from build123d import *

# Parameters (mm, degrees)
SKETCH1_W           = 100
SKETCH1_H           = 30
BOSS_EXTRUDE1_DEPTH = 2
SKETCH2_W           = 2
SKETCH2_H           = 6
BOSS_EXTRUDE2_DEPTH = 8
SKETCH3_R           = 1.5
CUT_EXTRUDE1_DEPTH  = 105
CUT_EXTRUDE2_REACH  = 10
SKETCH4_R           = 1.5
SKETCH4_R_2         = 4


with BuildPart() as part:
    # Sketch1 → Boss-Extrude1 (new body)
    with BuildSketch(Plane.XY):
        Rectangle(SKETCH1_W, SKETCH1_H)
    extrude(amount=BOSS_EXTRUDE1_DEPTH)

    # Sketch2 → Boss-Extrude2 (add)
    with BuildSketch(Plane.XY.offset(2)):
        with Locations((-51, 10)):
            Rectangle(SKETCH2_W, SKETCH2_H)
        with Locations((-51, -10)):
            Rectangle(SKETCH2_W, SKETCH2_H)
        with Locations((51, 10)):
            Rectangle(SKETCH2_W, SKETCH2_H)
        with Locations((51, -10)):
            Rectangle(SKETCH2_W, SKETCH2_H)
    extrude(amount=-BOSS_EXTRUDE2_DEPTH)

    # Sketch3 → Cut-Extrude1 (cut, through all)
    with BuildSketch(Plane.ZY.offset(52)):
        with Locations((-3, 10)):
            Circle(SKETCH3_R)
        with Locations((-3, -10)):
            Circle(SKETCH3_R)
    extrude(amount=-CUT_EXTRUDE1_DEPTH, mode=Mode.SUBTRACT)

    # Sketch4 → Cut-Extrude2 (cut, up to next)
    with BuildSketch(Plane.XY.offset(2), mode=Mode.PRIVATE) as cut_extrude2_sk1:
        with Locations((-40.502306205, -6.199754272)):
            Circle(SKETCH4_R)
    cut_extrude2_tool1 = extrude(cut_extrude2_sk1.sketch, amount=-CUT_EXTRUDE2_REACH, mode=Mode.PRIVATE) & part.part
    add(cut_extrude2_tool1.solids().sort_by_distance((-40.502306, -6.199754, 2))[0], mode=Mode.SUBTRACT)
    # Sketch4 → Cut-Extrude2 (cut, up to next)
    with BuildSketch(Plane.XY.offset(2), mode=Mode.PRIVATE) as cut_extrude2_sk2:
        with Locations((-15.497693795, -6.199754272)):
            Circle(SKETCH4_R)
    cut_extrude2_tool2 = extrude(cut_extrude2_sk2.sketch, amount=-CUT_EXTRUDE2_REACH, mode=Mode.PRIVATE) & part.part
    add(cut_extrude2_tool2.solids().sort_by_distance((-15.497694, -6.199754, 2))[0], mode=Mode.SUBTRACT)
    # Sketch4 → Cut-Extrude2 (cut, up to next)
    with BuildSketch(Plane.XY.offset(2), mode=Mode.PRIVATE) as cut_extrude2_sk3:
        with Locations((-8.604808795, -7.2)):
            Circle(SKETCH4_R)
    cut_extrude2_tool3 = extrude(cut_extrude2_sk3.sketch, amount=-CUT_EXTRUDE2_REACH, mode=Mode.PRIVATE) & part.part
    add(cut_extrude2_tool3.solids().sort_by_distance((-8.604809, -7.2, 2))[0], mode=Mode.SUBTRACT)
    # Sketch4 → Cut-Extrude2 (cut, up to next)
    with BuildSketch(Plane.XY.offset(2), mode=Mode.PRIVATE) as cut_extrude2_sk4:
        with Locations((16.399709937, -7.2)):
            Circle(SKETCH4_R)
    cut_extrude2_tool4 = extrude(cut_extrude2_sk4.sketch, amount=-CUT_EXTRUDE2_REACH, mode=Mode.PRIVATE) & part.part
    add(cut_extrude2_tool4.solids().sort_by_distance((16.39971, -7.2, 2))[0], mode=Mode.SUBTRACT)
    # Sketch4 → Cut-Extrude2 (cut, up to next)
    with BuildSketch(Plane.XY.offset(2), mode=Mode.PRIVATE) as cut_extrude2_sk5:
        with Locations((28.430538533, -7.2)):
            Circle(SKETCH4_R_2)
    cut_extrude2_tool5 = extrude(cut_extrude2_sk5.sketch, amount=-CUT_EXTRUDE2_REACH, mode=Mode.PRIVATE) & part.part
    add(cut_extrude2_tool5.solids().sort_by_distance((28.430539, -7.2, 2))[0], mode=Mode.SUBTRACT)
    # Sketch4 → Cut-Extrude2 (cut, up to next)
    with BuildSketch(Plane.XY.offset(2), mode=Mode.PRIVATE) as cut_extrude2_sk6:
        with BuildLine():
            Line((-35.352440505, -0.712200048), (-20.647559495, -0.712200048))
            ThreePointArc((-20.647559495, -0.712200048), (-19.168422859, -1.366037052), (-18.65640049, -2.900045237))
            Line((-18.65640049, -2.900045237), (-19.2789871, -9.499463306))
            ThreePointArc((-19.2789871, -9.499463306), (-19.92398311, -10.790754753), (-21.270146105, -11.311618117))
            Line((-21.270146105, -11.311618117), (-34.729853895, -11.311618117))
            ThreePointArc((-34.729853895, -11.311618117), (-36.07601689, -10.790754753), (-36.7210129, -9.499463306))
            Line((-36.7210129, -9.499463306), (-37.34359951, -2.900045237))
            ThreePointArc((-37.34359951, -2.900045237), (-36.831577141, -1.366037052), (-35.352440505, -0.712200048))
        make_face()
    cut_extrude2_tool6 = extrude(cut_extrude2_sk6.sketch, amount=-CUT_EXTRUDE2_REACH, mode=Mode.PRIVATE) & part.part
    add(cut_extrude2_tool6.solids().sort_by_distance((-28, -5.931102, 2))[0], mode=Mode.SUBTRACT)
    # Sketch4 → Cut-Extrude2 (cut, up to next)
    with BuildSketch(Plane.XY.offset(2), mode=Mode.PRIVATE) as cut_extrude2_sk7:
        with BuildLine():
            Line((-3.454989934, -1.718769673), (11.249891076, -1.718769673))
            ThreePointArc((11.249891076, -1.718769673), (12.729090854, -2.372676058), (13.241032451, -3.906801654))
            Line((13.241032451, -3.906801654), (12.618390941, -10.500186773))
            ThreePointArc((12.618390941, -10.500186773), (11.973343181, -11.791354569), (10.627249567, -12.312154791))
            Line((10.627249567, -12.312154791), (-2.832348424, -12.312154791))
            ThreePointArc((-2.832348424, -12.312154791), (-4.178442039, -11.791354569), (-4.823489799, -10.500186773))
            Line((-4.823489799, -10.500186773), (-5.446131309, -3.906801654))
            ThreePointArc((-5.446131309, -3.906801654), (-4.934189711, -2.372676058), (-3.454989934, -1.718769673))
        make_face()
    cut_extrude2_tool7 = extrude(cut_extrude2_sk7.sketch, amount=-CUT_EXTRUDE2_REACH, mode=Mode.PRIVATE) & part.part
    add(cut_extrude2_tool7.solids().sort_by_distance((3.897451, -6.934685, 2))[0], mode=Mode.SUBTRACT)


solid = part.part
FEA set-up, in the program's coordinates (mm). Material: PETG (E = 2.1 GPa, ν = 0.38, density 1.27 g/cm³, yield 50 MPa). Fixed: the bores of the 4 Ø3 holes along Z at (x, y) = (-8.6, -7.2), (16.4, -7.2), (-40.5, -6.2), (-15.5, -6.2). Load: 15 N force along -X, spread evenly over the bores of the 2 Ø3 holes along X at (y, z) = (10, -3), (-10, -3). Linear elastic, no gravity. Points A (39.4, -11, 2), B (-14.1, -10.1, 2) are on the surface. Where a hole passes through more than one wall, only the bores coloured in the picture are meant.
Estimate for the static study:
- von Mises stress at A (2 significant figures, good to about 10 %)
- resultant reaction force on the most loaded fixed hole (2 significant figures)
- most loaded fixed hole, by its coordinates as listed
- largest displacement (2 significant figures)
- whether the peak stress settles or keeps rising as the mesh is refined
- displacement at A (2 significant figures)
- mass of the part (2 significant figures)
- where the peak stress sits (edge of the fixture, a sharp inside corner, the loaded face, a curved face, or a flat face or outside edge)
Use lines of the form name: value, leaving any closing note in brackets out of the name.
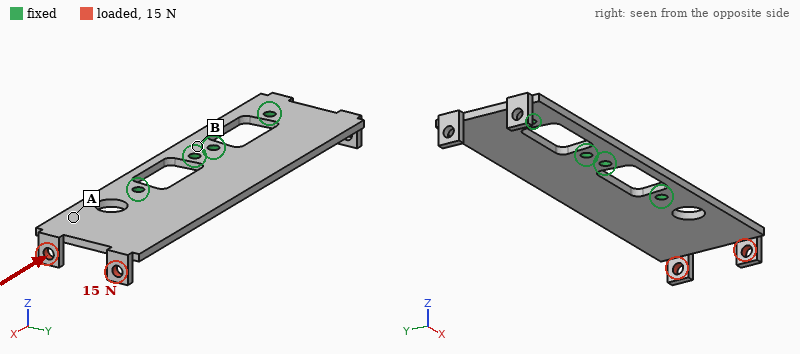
von Mises stress at A: 2.6 MPa
resultant reaction force on the most loaded fixed hole: 9.5 N
most loaded fixed hole, by its coordinates as listed: (16.4, -7.2)
largest displacement: 1.3 mm
whether the peak stress settles or keeps rising as the mesh is refined: keeps rising
displacement at A: 0.47 mm
mass of the part: 6.9 g
where the peak stress sits: edge of the fixture
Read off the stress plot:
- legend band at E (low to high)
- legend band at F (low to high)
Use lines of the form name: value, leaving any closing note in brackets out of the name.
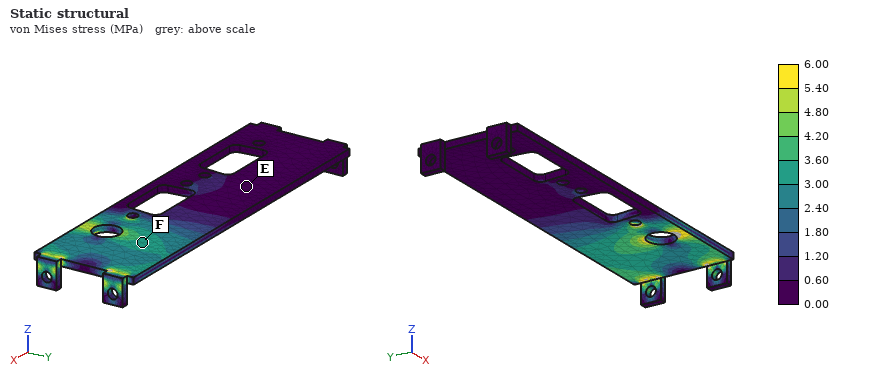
legend band at E: 0.00 to 0.60 MPa
legend band at F: 3.00 to 3.60 MPa
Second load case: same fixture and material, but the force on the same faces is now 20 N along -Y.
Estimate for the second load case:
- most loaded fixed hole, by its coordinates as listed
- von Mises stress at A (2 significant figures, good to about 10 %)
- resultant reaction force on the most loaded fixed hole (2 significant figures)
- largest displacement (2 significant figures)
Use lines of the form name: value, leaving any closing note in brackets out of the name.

most loaded fixed hole, by its coordinates as listed: (16.4, -7.2)
von Mises stress at A: 3.9 MPa
resultant reaction force on the most loaded fixed hole: 38 N
largest displacement: 1.1 mm
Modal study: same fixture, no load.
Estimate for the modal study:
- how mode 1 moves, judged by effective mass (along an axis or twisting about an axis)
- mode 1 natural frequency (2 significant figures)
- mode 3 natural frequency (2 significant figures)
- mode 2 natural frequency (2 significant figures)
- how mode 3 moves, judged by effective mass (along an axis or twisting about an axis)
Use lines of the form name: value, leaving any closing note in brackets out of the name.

how mode 1 moves, judged by effective mass: along Z
mode 1 natural frequency: 260 Hz
mode 3 natural frequency: 750 Hz
mode 2 natural frequency: 540 Hz
how mode 3 moves, judged by effective mass: along Z
